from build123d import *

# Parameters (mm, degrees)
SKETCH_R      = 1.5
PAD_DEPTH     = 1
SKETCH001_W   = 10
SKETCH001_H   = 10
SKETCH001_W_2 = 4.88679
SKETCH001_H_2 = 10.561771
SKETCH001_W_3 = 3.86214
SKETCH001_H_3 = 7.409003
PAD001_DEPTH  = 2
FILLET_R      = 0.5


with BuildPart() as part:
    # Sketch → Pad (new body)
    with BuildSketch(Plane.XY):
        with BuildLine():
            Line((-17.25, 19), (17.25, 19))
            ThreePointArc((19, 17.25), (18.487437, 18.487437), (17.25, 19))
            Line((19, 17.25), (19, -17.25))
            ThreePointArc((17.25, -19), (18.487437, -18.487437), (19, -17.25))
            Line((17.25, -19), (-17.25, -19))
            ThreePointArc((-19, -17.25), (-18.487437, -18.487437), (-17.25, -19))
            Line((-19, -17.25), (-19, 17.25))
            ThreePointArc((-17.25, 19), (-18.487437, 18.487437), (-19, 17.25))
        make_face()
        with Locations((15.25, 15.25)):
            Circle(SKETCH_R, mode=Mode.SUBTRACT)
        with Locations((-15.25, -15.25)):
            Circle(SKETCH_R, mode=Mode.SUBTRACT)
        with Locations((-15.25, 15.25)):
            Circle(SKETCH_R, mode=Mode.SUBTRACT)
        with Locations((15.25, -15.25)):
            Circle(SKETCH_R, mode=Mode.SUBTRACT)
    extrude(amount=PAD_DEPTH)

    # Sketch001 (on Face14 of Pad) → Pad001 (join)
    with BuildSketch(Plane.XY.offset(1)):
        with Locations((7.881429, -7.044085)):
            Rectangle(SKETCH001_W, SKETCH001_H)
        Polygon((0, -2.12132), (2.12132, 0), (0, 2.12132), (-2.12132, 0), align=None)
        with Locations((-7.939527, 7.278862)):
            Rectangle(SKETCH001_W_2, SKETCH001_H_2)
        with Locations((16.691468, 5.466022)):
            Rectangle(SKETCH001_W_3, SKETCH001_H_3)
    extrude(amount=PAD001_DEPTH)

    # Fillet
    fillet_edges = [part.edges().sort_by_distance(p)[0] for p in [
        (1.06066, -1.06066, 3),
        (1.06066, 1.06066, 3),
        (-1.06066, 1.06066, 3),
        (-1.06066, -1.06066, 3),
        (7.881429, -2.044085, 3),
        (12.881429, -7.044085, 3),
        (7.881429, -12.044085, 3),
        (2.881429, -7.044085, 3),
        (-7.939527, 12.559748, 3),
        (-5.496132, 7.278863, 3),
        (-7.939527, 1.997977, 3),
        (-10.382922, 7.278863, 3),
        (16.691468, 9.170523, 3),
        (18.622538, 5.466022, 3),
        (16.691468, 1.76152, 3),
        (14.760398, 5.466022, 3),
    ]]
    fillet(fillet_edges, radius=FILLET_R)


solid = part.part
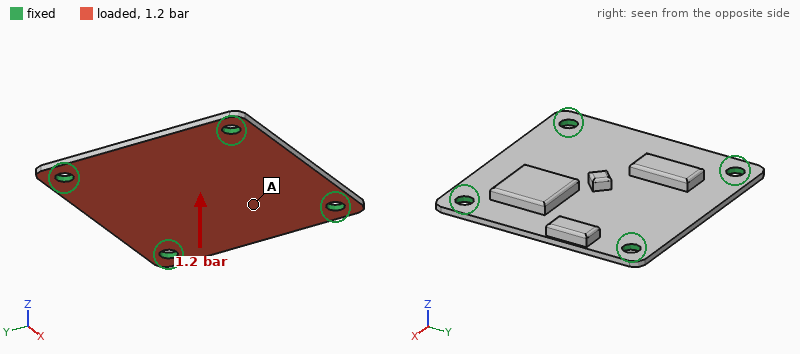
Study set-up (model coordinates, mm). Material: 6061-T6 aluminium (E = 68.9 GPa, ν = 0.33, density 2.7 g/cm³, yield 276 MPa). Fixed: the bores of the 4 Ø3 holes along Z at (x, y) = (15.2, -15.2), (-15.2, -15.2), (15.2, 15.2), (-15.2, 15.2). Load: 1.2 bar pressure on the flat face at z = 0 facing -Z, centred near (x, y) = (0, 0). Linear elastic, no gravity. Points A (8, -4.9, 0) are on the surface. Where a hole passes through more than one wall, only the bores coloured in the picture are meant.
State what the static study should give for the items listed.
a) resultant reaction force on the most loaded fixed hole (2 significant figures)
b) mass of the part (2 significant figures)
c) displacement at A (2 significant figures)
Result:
47 N
4.8 g
54 µm
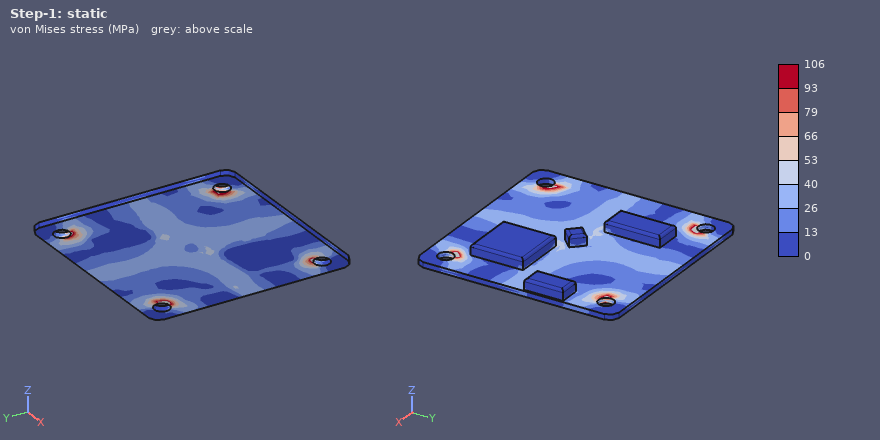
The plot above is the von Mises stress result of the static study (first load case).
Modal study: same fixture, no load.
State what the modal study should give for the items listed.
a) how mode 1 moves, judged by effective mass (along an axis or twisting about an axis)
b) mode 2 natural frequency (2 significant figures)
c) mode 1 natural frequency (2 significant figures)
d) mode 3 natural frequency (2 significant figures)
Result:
along Z
6700 Hz
3900 Hz
7400 Hz
